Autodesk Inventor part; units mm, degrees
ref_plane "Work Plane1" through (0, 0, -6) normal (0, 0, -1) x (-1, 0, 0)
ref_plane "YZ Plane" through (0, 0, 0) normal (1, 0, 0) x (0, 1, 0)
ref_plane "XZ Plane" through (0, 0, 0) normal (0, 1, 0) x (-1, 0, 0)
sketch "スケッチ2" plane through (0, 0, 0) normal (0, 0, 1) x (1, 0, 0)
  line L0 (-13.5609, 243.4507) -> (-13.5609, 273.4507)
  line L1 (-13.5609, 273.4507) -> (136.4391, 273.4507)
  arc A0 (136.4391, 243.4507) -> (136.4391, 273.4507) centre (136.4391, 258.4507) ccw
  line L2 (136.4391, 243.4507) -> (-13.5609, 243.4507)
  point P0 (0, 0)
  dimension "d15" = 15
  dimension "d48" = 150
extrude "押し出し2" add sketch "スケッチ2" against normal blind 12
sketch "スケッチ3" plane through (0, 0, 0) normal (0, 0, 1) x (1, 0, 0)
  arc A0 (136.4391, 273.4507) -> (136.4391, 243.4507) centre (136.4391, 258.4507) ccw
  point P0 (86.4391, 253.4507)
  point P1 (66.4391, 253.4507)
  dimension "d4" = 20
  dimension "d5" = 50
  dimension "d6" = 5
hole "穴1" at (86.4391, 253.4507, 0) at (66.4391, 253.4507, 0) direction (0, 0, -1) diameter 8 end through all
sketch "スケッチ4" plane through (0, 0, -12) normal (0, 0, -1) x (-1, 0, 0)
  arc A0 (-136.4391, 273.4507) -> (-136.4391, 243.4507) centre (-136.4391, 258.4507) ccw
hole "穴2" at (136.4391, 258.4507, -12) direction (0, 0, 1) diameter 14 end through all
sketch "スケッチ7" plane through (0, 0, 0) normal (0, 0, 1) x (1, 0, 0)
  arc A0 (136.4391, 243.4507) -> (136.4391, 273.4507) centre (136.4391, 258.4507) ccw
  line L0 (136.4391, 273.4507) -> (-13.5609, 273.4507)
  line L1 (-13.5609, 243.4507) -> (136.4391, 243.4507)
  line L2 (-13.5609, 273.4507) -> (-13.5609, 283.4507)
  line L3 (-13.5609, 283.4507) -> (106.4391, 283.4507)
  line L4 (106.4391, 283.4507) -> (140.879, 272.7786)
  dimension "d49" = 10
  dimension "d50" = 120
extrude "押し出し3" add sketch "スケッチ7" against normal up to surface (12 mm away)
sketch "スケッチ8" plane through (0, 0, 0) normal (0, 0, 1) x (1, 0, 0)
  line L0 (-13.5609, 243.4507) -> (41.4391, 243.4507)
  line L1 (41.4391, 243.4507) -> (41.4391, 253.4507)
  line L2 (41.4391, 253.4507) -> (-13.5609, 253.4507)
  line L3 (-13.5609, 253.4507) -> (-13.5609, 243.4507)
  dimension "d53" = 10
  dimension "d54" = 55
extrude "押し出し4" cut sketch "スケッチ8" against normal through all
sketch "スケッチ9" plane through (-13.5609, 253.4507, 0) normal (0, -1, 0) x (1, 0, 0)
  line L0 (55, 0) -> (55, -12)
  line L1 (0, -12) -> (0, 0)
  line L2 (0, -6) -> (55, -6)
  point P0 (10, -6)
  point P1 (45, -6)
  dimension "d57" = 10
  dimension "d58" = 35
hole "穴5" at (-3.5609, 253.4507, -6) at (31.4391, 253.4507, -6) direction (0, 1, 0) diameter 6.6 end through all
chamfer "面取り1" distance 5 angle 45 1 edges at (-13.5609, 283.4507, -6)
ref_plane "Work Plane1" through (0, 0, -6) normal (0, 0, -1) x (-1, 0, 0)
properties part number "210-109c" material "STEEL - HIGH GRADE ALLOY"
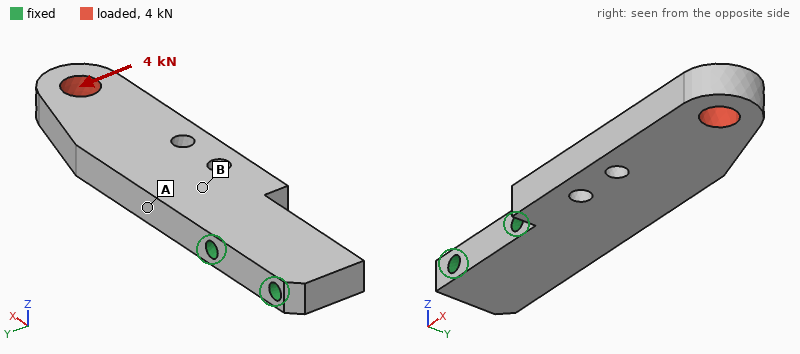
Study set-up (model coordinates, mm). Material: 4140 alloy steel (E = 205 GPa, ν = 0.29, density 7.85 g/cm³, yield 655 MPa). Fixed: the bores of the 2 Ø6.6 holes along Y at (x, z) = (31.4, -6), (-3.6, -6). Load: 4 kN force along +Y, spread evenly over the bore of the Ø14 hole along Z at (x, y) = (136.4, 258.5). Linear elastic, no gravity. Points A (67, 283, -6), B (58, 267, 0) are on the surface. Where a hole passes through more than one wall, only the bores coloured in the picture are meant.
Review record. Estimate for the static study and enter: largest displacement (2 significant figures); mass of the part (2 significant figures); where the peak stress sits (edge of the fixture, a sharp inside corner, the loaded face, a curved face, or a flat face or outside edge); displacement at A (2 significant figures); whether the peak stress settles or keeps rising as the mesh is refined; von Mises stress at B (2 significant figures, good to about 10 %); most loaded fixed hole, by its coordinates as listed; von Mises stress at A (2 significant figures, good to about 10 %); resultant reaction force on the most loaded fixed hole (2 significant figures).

0.24 mm
490 g
edge of the fixture
0.048 mm
keeps rising
40 MPa
(31.4, -6)
100 MPa
4.2 kN
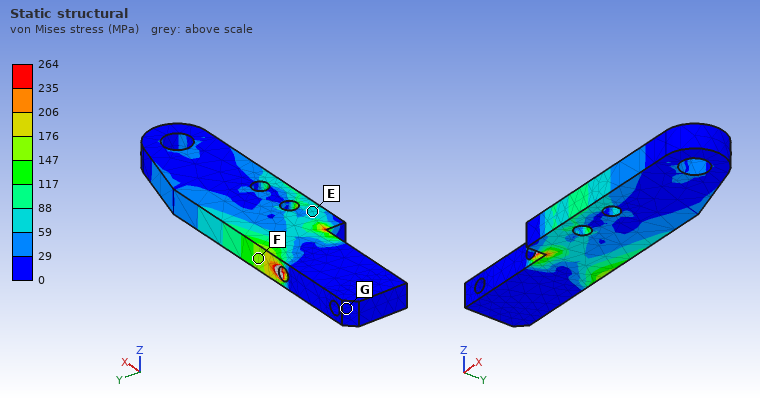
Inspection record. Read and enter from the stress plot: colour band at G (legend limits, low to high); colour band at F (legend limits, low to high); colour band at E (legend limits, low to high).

0 to 29 MPa
147 to 176 MPa
59 to 88 MPa
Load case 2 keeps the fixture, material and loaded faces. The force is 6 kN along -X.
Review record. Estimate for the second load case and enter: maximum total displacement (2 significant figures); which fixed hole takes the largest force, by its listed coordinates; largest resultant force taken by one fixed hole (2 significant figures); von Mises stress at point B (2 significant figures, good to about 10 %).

38 µm
(31.4, -6)
5.9 kN
18 MPa
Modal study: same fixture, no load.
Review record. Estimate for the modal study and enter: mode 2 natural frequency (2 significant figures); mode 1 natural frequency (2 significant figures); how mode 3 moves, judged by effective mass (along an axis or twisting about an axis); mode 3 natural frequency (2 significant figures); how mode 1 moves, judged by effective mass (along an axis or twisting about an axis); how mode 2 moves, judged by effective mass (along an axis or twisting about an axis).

2000 Hz
760 Hz
twisting about X
4000 Hz
along Z
along Y
